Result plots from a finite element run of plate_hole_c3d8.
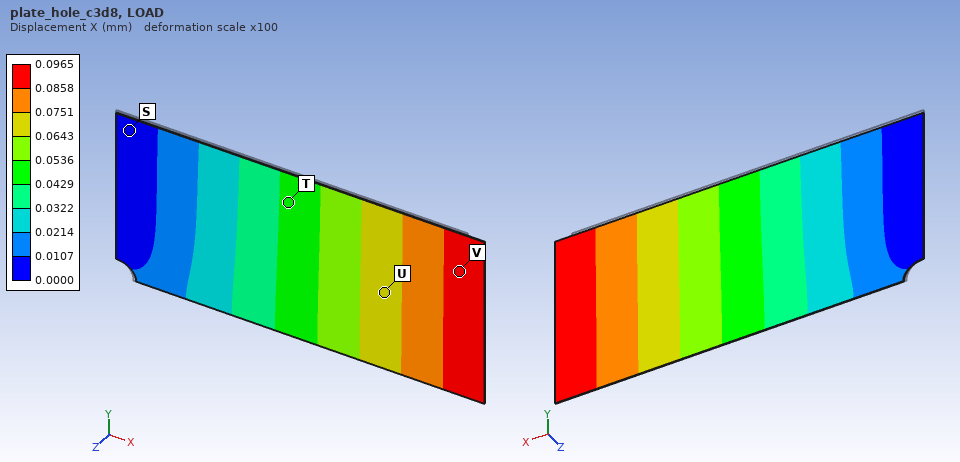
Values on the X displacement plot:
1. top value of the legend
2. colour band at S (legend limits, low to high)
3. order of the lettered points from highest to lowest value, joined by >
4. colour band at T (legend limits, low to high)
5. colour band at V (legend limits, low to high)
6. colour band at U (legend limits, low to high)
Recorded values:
0.0965 mm
0.0000 to 0.0107 mm
V > U > T > S
0.0429 to 0.0536 mm
0.0858 to 0.0965 mm
0.0643 to 0.0751 mm
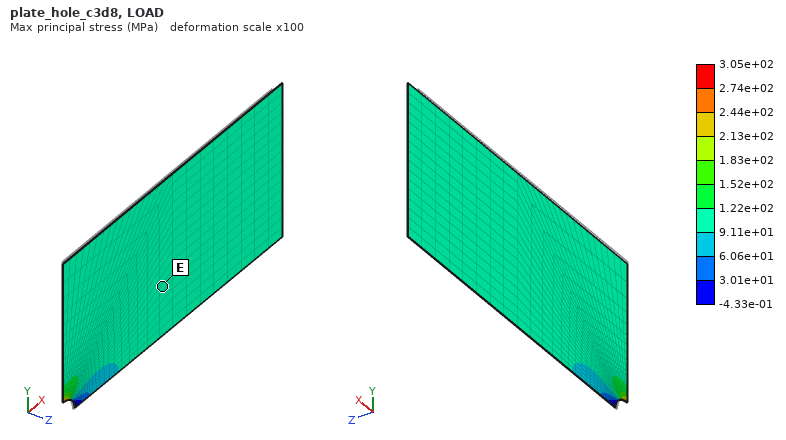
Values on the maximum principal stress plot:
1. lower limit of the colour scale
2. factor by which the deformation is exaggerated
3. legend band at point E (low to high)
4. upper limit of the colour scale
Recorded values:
-4.33e-01 MPa
100
9.11e+01 to 1.22e+02 MPa
3.05e+02 MPa
